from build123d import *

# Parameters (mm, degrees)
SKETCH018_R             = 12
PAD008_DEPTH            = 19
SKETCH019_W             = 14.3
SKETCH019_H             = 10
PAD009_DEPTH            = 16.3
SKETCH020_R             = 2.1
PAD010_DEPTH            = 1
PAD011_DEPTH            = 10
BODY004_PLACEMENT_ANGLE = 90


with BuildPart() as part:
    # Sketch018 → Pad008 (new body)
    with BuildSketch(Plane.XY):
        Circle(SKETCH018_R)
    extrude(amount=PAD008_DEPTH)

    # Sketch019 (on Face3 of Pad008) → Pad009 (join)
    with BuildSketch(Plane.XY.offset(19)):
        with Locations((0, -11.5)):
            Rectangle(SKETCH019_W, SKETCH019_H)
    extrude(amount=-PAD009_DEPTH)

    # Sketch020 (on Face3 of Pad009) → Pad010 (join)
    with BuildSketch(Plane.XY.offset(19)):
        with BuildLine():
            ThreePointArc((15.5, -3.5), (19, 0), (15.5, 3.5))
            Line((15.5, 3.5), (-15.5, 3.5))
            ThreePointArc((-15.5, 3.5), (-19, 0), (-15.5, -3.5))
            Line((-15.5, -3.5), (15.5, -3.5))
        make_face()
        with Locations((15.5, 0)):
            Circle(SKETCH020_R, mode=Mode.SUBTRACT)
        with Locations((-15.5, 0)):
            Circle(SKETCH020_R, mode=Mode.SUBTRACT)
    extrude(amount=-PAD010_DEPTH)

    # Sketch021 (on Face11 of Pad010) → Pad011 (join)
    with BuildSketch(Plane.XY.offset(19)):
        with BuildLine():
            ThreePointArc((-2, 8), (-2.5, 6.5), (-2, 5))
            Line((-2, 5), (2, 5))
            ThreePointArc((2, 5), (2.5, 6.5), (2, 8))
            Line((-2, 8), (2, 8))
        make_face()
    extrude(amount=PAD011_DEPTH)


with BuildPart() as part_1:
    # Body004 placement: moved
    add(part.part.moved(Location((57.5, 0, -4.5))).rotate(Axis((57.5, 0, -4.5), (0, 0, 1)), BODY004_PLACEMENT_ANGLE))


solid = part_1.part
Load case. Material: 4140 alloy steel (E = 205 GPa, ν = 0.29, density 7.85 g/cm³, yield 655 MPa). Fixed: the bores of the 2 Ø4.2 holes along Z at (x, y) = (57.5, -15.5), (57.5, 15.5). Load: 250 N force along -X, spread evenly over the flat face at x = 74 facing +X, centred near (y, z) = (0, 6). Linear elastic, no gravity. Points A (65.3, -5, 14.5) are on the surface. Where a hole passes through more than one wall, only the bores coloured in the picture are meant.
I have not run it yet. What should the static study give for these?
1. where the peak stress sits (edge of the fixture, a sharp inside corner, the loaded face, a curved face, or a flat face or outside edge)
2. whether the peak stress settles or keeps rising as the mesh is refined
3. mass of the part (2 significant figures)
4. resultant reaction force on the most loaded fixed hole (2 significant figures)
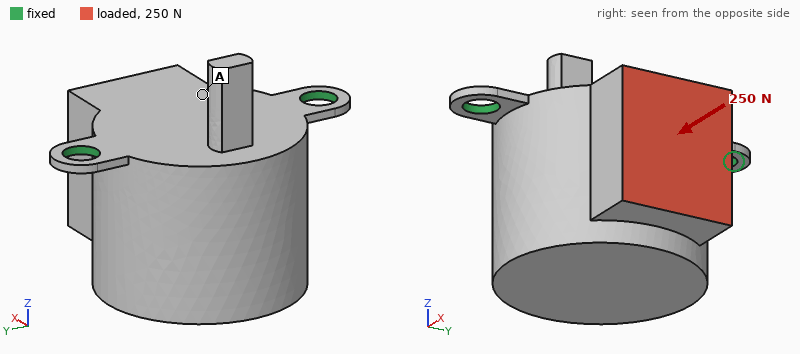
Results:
edge of the fixture
keeps rising
79 g
130 N
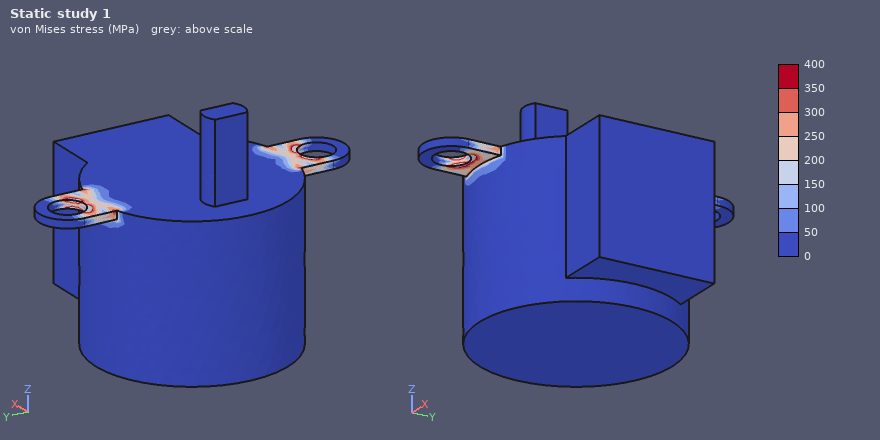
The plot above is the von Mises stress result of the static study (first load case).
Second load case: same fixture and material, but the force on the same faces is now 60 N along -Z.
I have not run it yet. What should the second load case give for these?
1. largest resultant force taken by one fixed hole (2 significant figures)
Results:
35 N
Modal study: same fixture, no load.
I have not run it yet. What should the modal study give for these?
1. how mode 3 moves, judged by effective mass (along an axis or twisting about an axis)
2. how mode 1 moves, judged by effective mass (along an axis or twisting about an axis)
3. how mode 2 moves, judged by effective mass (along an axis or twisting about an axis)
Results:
along Y
along X
along Z
